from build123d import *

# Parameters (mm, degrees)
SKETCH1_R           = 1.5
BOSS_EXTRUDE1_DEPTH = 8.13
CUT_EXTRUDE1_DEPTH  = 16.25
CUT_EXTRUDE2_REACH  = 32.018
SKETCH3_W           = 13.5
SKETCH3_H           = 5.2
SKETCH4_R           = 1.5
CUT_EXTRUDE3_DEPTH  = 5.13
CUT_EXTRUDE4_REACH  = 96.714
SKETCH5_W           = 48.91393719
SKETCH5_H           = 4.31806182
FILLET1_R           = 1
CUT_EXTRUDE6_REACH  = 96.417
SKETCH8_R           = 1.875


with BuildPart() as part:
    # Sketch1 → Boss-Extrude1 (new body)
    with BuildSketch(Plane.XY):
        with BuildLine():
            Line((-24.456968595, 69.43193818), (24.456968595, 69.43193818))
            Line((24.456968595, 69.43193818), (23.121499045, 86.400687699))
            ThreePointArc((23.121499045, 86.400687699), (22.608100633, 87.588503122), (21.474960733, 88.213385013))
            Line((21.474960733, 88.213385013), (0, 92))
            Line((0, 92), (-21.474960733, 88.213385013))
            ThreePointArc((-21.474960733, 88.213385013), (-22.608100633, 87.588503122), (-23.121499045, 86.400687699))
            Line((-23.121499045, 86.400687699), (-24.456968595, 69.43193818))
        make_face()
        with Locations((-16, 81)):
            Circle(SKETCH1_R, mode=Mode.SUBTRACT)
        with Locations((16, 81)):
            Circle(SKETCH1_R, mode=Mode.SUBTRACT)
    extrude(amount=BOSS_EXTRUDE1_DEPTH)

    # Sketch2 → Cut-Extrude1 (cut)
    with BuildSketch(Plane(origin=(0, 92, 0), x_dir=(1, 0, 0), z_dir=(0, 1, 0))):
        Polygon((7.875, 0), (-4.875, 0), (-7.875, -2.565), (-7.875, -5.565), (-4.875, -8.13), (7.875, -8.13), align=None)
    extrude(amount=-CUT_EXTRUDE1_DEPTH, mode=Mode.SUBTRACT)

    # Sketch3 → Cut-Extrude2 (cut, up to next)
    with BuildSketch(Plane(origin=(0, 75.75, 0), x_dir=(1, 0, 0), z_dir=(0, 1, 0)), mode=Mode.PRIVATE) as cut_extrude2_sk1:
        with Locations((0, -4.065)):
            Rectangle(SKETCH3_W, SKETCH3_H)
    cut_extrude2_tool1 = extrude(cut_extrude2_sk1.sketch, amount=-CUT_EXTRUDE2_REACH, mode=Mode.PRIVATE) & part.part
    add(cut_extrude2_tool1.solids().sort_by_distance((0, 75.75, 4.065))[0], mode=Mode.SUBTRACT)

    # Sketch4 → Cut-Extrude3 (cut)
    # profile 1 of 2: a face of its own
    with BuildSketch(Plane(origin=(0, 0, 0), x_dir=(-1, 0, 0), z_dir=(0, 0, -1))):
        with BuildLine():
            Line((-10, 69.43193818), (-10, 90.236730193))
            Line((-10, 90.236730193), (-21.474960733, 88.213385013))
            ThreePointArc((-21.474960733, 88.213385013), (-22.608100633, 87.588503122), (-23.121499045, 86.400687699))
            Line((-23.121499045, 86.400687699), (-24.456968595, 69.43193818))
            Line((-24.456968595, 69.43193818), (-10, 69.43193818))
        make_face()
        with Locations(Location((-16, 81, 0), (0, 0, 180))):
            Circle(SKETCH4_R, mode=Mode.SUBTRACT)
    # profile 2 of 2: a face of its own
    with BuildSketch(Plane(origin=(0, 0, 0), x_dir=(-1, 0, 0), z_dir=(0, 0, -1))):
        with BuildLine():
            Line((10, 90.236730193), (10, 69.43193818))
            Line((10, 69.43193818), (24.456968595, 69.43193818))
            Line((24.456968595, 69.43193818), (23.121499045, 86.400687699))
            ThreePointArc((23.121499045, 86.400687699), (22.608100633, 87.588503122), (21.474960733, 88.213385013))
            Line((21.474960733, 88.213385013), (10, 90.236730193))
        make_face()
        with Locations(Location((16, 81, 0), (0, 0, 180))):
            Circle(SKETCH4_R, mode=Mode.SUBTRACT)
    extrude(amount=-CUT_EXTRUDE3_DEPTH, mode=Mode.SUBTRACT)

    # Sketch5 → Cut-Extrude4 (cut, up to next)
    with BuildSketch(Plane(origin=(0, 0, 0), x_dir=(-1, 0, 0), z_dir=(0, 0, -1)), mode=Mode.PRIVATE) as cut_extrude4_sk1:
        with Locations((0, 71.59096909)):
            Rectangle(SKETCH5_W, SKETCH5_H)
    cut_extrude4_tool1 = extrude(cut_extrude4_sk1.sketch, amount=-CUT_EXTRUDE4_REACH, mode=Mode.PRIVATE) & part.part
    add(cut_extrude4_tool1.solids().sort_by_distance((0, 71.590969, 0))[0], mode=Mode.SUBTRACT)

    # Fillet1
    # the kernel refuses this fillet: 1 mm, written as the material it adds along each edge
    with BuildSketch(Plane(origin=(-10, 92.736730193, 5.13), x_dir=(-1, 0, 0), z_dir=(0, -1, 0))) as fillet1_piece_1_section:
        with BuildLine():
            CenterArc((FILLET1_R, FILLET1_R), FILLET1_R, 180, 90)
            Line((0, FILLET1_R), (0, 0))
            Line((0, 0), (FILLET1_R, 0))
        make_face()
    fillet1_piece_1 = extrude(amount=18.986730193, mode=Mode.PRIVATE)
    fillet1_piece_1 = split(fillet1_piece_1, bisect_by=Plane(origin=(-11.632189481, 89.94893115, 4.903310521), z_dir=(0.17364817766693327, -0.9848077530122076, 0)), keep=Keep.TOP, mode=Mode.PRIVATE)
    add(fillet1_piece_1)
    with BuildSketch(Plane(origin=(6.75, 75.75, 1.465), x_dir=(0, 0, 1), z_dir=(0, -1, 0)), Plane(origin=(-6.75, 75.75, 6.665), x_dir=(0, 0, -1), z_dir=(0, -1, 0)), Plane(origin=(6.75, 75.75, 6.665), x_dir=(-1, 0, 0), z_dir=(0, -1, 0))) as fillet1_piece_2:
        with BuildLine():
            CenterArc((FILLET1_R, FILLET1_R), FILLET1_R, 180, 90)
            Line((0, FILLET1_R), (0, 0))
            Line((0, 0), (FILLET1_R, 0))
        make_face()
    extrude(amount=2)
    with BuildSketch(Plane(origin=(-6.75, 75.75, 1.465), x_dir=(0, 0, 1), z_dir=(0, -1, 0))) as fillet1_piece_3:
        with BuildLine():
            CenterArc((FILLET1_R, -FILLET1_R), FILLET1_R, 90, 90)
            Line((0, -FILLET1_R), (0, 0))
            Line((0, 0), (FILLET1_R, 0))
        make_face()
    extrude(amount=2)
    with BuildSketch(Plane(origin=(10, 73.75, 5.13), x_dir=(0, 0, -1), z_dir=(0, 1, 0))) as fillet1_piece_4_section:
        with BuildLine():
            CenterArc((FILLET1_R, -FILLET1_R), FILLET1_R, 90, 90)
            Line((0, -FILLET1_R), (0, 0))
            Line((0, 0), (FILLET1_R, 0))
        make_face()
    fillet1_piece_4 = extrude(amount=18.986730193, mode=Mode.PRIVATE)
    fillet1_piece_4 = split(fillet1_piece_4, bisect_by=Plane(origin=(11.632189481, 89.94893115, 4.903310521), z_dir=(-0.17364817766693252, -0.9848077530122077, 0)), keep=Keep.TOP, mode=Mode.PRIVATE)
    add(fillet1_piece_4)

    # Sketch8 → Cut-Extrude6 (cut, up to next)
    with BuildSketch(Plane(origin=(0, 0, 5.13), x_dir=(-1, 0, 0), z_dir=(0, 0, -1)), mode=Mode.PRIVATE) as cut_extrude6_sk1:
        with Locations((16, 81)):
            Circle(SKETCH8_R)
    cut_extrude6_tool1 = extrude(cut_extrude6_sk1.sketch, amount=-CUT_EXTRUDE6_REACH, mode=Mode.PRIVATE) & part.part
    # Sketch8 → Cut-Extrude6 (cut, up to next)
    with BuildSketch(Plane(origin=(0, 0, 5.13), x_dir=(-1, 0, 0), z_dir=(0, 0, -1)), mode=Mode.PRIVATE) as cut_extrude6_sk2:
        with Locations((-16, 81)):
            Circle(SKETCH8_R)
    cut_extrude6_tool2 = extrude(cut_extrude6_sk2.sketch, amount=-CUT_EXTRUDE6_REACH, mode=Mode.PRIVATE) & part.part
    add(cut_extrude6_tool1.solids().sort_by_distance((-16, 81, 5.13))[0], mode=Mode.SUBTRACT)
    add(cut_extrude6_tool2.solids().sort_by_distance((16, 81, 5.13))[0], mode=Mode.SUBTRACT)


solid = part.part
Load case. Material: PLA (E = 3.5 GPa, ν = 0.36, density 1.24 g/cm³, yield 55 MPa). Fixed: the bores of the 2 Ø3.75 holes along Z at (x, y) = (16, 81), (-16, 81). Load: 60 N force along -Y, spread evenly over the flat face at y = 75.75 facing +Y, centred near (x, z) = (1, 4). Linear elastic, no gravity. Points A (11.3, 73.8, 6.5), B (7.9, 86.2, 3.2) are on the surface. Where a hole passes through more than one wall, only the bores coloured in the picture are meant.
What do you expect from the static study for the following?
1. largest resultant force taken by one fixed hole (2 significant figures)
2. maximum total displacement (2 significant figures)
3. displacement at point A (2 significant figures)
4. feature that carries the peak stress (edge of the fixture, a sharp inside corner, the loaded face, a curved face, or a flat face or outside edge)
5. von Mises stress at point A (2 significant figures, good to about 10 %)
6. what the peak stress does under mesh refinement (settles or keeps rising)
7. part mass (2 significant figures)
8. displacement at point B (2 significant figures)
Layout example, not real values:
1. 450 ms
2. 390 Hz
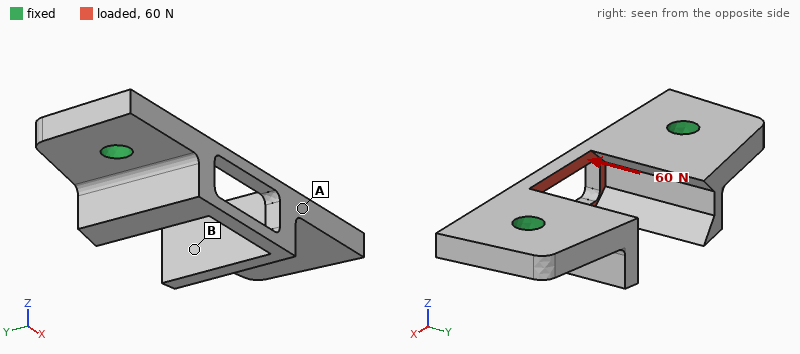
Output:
1. 36 N
2. 0.12 mm
3. 0.018 mm
4. a sharp inside corner
5. 3.6 MPa
6. keeps rising
7. 2.5 g
8. 0.021 mm
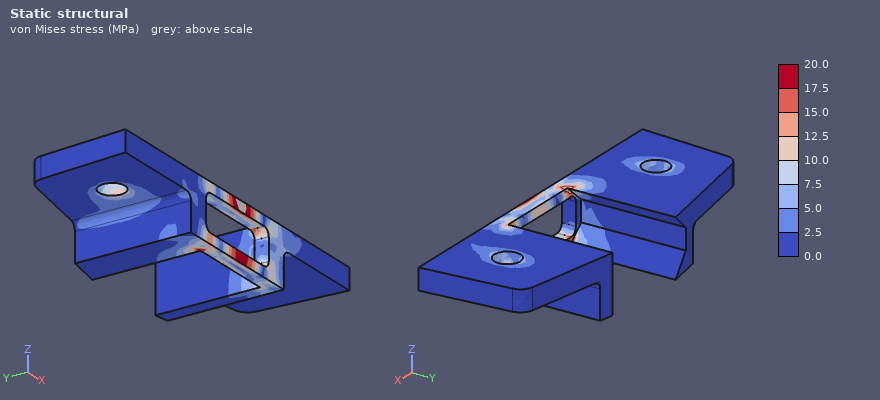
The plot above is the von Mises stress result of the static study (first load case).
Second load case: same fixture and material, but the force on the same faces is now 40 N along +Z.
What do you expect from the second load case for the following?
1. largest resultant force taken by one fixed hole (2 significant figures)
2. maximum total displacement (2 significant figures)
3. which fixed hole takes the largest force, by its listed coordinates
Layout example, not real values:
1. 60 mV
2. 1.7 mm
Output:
1. 23 N
2. 0.13 mm
3. (16, 81)
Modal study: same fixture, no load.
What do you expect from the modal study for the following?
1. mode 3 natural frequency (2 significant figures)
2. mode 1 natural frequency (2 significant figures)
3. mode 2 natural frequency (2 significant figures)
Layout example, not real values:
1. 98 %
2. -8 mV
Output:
1. 6500 Hz
2. 5100 Hz
3. 5900 Hz
